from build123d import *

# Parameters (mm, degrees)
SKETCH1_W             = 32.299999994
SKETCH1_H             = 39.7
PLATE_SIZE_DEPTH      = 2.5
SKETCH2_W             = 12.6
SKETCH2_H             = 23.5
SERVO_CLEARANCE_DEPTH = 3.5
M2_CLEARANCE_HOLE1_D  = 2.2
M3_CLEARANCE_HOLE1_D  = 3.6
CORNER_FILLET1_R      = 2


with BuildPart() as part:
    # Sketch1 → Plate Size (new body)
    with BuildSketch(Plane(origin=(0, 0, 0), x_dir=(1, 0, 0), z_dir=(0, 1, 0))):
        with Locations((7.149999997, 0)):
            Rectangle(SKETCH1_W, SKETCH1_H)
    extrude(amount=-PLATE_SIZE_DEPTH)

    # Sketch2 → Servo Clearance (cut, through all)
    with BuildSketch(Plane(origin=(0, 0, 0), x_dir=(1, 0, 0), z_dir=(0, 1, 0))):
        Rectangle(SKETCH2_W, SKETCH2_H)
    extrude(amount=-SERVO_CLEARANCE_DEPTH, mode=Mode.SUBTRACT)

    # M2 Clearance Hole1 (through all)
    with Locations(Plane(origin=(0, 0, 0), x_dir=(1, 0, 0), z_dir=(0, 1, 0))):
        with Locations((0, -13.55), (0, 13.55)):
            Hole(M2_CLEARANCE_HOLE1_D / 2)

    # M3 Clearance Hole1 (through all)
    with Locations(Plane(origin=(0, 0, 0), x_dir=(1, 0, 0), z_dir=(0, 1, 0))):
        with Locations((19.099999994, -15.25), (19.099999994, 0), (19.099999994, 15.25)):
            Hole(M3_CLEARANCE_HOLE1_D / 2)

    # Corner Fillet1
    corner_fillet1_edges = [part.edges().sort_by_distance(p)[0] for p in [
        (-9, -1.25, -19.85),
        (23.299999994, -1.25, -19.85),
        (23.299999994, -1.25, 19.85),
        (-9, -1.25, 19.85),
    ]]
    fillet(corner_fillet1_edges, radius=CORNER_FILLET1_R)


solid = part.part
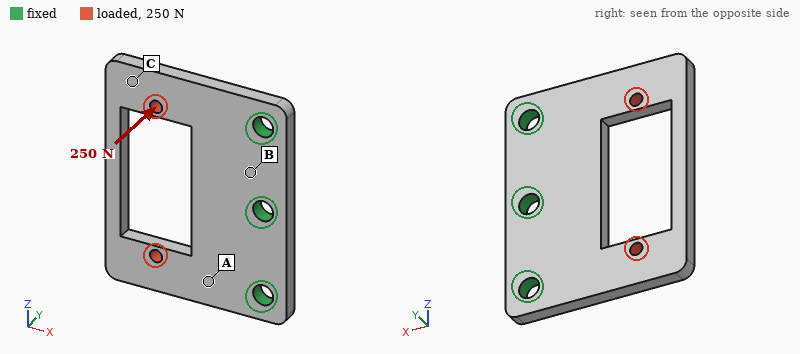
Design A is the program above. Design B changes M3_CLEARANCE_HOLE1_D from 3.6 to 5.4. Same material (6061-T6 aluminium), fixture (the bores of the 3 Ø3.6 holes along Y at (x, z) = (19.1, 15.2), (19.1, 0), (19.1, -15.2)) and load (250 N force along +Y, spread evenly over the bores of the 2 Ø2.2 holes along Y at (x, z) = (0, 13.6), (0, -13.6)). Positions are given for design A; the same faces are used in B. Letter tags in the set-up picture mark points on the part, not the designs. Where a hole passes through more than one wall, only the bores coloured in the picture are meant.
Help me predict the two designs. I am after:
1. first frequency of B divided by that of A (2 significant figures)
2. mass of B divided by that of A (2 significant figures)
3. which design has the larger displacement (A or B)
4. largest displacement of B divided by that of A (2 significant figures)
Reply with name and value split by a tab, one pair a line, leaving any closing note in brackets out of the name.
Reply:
first frequency of B divided by that of A	1.1
mass of B divided by that of A	0.96
which design has the larger displacement	A
largest displacement of B divided by that of A	0.89
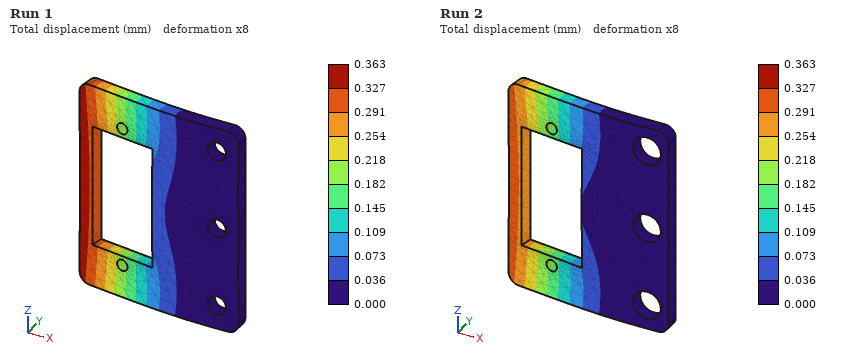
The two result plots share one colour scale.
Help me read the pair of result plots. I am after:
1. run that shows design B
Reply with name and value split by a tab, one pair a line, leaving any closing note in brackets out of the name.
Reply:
run that shows design B	Run 2
